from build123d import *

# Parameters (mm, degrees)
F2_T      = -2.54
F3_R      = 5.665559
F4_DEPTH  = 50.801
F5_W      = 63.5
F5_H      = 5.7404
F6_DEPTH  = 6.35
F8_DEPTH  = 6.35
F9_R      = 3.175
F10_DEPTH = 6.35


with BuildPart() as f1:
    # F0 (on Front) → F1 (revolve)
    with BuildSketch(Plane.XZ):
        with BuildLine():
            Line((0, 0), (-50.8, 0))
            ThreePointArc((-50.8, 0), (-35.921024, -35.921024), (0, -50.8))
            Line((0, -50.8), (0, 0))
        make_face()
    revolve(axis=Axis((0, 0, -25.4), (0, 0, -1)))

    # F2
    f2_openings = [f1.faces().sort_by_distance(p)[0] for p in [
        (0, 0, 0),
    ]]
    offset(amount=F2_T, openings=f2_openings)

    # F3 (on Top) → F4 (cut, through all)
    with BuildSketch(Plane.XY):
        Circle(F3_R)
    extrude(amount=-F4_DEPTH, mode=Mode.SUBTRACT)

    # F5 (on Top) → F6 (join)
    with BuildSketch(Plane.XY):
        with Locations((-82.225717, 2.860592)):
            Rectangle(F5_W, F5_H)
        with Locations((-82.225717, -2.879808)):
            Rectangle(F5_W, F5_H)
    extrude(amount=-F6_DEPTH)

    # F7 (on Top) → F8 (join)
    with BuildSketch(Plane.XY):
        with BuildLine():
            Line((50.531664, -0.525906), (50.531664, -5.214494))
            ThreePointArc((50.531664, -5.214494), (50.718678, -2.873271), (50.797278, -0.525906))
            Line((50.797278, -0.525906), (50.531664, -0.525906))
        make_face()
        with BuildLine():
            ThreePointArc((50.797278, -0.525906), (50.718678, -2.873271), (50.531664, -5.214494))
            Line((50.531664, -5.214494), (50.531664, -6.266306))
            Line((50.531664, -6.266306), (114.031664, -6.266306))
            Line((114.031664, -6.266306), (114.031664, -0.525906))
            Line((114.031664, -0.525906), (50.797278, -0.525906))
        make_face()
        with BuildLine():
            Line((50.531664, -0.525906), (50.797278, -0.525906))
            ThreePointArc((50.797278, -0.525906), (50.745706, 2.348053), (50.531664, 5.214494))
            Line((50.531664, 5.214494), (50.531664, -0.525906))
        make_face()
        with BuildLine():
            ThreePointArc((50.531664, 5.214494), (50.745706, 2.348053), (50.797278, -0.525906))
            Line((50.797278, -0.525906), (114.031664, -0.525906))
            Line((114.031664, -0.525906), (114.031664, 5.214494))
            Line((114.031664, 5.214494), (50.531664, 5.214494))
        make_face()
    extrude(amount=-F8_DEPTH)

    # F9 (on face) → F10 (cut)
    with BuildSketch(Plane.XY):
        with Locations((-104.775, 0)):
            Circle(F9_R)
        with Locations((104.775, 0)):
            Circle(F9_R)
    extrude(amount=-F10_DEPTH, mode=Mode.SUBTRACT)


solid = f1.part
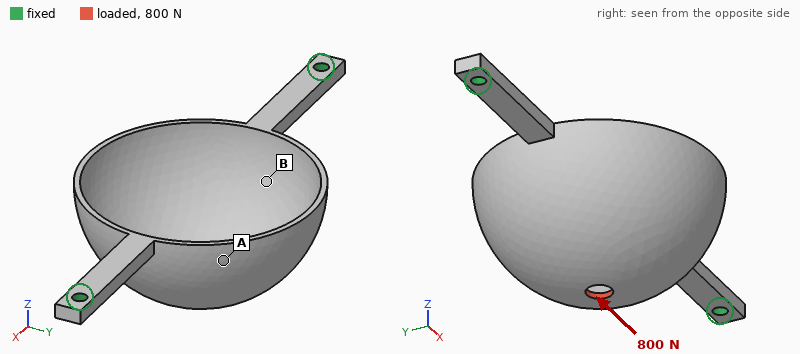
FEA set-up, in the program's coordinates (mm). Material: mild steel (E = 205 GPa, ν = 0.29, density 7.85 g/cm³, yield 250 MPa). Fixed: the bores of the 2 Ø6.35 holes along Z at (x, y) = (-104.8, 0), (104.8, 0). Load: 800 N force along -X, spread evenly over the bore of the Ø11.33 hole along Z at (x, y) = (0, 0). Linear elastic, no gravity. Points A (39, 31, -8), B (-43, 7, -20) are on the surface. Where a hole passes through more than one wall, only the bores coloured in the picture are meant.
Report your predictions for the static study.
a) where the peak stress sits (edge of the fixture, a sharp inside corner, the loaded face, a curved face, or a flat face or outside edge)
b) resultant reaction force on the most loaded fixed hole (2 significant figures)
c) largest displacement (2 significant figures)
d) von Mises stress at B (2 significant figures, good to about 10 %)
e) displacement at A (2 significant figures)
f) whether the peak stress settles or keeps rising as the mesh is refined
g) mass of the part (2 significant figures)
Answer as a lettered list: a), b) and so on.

a) a sharp inside corner
b) 480 N
c) 0.11 mm
d) 24 MPa
e) 0.088 mm
f) keeps rising
g) 370 g
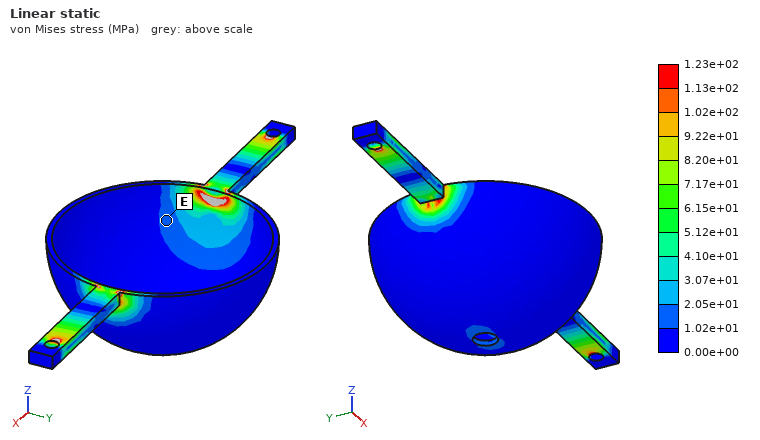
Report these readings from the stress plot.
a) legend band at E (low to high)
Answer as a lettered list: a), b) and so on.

a) 1.02e+01 to 2.05e+01 MPa
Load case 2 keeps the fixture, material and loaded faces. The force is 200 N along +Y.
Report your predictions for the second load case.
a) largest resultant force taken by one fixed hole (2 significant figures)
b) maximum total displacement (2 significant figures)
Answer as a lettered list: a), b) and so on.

a) 100 N
b) 0.29 mm
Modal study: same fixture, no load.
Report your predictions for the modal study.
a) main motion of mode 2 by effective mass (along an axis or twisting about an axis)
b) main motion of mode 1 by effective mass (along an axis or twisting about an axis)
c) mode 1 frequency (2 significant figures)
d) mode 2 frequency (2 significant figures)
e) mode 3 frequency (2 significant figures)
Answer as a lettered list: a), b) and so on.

a) along Z
b) along Y
c) 300 Hz
d) 540 Hz
e) 890 Hz
